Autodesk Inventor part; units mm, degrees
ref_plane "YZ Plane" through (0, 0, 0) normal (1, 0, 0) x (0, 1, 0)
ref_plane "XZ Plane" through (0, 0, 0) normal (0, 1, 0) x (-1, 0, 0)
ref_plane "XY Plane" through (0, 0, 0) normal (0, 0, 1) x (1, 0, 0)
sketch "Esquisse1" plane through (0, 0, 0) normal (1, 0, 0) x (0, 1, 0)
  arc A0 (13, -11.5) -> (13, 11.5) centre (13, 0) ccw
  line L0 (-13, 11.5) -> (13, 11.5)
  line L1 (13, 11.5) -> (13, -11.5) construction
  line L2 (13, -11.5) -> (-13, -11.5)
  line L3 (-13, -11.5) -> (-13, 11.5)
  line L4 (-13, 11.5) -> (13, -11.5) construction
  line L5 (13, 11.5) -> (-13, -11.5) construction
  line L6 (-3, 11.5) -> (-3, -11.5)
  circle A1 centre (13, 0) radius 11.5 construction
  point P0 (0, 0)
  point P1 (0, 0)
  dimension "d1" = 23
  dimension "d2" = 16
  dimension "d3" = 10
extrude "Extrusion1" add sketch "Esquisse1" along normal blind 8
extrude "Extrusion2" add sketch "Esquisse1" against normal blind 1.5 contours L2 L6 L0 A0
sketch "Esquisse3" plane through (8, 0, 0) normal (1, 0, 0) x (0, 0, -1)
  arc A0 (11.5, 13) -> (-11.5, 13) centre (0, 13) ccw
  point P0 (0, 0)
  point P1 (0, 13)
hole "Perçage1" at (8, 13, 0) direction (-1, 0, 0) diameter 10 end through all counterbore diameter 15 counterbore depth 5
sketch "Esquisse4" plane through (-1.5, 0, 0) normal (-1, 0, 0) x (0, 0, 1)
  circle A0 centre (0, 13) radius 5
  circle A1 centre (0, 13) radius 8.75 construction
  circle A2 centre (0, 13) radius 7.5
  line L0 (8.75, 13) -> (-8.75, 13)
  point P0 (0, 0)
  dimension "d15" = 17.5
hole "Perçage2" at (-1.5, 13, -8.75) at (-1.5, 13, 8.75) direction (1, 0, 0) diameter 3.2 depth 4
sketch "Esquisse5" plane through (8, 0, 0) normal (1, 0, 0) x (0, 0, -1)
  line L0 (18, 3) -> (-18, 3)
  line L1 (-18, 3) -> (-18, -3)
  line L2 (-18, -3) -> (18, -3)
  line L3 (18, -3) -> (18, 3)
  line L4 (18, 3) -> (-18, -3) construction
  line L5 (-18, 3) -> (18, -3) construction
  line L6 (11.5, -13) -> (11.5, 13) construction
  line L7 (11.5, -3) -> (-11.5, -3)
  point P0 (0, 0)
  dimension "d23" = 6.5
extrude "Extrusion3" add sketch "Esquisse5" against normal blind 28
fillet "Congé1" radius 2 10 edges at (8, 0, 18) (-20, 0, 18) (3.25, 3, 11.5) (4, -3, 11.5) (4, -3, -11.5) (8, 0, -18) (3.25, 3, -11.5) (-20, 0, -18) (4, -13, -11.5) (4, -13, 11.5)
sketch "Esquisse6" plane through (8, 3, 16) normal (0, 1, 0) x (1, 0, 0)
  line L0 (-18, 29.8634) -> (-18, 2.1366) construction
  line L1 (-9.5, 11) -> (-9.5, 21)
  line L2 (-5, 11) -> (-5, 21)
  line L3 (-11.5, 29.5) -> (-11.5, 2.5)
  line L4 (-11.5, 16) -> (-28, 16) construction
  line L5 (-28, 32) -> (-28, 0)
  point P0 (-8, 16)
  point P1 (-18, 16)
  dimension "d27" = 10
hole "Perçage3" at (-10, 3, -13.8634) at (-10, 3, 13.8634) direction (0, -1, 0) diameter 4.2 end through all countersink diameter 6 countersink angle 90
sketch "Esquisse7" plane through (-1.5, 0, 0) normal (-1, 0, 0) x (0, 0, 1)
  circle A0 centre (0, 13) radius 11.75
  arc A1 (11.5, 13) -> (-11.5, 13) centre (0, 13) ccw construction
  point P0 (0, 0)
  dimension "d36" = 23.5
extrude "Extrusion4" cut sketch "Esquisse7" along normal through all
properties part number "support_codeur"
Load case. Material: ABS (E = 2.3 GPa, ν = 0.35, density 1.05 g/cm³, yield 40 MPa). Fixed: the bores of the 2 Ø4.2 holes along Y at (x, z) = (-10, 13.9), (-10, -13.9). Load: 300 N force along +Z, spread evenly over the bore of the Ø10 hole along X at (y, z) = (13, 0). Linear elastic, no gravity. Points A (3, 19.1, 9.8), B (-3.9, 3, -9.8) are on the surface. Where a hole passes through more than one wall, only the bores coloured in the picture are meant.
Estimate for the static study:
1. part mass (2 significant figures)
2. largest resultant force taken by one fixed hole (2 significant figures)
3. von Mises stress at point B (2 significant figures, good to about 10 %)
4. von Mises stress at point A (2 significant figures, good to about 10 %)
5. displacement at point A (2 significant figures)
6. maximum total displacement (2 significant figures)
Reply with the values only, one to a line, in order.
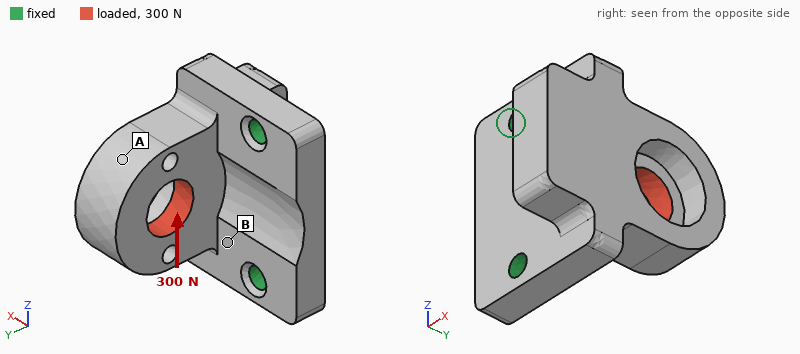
11 g
230 N
8.4 MPa
2.7 MPa
0.25 mm
0.29 mm
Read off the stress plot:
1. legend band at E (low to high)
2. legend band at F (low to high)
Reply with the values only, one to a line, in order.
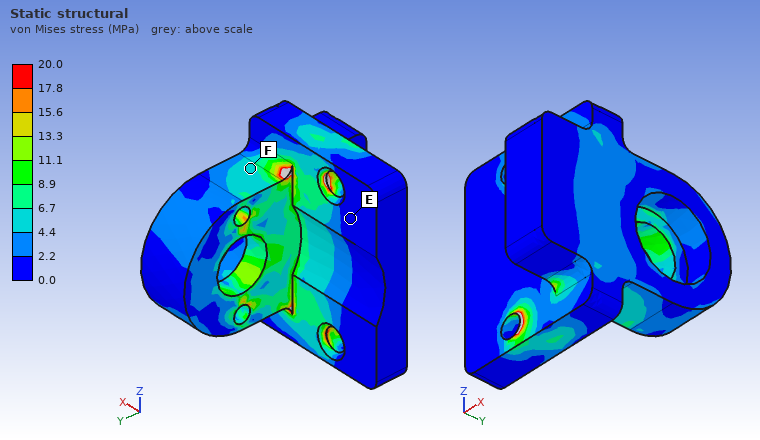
0.0 to 2.2 MPa
4.4 to 6.7 MPa
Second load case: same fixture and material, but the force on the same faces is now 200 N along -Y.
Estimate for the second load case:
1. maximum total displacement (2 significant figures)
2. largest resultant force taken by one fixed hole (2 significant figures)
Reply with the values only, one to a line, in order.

0.28 mm
100 N
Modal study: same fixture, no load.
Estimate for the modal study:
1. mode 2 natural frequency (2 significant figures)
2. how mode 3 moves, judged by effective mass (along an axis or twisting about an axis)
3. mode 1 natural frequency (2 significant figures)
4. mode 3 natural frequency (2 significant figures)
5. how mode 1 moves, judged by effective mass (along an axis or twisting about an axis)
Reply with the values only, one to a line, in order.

3200 Hz
along Y
1400 Hz
4000 Hz
along Y
